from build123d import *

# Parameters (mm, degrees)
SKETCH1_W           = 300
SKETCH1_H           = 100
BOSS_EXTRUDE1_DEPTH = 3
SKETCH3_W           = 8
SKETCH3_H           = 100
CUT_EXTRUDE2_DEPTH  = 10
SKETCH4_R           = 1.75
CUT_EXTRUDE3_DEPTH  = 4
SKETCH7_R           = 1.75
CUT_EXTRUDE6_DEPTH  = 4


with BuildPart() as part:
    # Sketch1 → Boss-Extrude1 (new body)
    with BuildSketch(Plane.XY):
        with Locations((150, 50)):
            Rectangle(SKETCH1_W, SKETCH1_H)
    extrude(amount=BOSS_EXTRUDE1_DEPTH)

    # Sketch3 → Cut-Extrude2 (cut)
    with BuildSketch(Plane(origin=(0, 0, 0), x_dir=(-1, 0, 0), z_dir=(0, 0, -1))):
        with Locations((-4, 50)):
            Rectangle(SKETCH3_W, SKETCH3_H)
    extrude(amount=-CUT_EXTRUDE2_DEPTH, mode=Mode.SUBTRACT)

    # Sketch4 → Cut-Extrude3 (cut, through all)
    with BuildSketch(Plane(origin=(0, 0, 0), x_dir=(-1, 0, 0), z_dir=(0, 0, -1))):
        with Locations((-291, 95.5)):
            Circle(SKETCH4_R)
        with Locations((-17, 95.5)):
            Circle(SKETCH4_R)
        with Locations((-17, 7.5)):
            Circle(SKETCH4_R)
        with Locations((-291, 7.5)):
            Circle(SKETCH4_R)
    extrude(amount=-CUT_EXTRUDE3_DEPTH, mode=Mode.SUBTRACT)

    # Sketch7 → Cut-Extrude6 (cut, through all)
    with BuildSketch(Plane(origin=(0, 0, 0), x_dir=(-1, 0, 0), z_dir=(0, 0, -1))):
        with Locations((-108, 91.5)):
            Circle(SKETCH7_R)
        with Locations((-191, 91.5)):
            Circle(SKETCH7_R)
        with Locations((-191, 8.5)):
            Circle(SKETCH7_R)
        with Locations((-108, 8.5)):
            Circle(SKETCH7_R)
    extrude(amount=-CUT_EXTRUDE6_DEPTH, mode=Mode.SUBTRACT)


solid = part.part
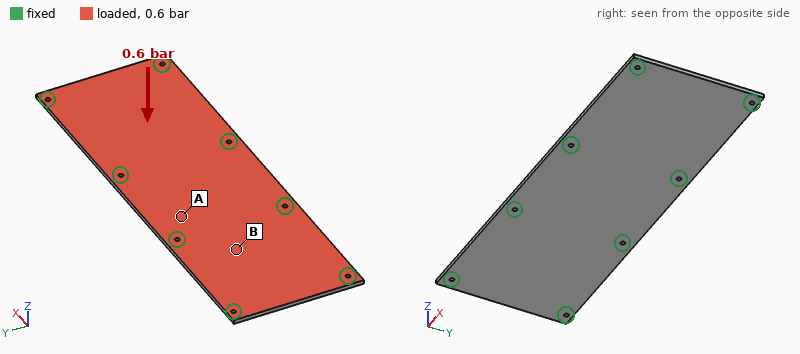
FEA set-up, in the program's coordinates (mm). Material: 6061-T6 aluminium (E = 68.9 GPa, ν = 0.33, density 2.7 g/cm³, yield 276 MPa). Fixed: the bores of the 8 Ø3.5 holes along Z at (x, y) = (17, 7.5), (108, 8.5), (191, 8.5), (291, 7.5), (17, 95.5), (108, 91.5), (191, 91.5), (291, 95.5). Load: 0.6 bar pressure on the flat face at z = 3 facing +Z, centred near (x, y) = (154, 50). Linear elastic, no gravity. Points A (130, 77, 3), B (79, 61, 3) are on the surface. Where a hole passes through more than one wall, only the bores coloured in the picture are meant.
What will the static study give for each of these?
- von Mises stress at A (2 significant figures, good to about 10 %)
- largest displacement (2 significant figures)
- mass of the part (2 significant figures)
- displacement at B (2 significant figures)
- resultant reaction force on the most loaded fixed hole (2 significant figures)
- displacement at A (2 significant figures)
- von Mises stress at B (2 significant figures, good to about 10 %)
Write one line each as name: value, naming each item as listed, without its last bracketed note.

von Mises stress at A: 6.7 MPa
largest displacement: 0.20 mm
mass of the part: 240 g
displacement at B: 0.14 mm
resultant reaction force on the most loaded fixed hole: 280 N
displacement at A: 0.062 mm
von Mises stress at B: 13 MPa
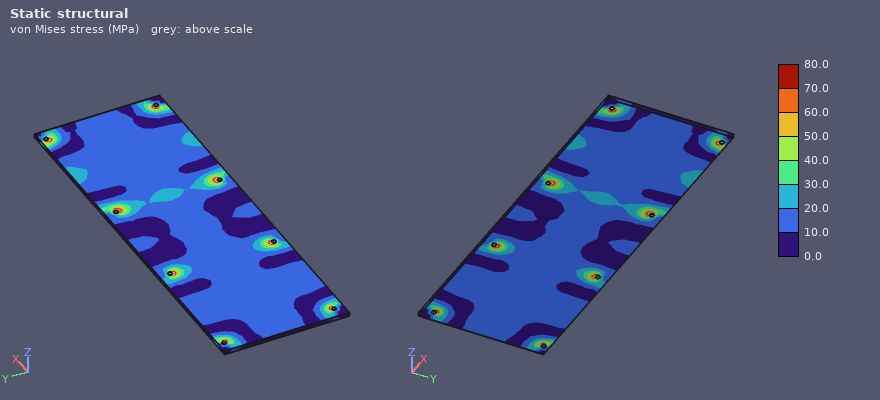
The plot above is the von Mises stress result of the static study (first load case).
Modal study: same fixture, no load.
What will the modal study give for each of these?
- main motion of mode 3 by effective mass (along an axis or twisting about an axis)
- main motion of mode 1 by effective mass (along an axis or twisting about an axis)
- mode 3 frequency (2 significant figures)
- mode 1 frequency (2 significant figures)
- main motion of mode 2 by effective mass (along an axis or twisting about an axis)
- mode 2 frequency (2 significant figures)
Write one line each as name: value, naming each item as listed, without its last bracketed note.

main motion of mode 3 by effective mass: along Z
main motion of mode 1 by effective mass: along Z
mode 3 frequency: 1500 Hz
mode 1 frequency: 1100 Hz
main motion of mode 2 by effective mass: along Z
mode 2 frequency: 1300 Hz
